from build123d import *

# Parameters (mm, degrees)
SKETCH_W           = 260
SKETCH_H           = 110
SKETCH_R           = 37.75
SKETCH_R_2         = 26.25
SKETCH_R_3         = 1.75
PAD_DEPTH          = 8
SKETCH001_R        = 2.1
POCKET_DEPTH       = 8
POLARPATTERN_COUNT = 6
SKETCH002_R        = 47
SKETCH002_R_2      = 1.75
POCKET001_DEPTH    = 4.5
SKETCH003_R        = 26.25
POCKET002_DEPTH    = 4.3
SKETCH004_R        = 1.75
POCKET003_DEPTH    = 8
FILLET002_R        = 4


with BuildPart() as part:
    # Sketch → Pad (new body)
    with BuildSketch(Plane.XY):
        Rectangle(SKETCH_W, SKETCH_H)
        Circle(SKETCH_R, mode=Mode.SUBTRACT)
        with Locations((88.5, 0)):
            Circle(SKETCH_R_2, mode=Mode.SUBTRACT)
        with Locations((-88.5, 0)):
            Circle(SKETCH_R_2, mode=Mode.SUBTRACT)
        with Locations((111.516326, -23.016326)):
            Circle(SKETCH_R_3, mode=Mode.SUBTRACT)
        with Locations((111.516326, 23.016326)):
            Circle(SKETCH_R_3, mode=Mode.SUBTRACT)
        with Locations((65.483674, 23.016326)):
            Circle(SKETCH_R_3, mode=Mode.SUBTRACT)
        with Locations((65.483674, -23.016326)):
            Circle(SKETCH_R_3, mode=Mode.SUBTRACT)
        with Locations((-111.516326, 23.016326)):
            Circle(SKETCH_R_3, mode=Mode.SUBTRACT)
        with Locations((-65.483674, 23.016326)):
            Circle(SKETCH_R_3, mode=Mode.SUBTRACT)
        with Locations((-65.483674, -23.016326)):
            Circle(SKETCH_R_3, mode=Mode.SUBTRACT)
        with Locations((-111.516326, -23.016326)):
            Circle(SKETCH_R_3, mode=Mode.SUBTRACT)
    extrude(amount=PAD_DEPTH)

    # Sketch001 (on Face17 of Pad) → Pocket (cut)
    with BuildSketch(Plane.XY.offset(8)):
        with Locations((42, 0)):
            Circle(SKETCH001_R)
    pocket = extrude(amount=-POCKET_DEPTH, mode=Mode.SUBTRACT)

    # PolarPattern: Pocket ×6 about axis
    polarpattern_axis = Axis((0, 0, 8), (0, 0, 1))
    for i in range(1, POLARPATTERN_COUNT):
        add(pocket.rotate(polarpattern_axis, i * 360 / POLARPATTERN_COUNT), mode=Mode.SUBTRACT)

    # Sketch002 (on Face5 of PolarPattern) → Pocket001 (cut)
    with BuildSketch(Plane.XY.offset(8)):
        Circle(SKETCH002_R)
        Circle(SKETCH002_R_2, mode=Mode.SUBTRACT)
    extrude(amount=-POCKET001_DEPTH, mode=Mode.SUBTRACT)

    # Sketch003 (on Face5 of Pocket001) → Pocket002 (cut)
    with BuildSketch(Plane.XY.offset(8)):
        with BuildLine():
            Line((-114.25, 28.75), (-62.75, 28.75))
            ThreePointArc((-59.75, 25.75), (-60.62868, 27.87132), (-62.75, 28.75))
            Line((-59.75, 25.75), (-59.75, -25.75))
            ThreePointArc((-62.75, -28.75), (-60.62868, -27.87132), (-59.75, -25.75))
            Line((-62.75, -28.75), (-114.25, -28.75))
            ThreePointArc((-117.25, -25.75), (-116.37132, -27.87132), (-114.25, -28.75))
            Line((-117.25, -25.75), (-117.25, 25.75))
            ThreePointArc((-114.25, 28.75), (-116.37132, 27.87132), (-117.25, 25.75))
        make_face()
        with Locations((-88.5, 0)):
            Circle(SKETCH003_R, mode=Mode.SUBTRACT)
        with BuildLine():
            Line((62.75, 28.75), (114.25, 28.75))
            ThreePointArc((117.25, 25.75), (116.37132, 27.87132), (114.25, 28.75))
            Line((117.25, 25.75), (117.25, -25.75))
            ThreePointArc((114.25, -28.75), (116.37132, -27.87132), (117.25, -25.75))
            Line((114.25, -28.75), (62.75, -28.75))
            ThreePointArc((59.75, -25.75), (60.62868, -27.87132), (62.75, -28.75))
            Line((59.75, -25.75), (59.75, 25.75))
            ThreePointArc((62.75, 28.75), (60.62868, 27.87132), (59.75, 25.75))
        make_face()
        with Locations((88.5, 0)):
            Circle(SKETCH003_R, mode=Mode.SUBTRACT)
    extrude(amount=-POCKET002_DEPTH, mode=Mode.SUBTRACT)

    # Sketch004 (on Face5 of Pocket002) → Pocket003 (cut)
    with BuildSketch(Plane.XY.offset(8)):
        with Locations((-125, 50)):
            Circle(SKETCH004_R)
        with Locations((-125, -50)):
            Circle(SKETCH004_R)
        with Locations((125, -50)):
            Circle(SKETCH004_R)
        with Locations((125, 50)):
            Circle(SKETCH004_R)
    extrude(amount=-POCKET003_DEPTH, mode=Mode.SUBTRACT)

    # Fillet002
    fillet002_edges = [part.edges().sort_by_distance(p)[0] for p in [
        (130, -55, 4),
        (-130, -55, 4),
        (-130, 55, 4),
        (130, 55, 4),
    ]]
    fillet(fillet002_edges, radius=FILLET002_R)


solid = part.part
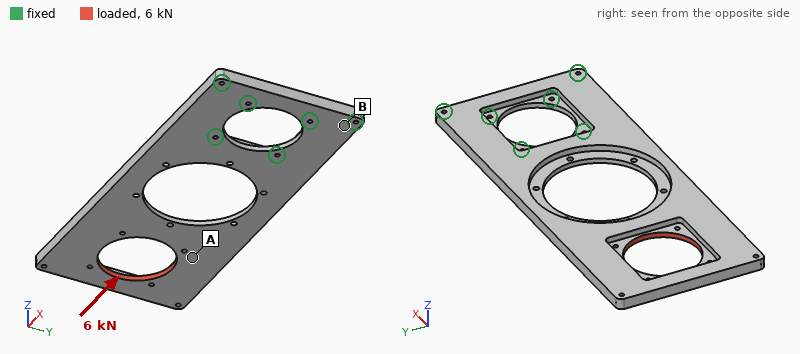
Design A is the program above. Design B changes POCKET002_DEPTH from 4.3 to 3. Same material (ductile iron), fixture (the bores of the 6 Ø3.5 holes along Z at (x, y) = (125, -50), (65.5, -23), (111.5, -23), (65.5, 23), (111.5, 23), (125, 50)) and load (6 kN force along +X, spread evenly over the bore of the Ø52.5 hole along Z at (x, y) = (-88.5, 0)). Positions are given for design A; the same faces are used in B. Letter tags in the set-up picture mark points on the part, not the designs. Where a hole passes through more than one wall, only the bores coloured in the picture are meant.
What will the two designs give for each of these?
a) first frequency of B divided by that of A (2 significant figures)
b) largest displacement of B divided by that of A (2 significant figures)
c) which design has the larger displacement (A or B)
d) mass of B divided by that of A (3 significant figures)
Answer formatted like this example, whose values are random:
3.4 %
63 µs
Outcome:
1.0
0.59
A
1.02
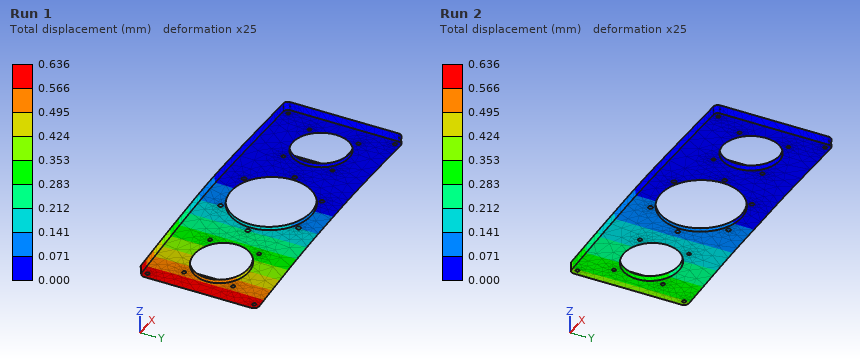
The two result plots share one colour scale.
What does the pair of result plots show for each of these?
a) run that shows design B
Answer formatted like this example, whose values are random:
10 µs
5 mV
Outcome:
Run 2
